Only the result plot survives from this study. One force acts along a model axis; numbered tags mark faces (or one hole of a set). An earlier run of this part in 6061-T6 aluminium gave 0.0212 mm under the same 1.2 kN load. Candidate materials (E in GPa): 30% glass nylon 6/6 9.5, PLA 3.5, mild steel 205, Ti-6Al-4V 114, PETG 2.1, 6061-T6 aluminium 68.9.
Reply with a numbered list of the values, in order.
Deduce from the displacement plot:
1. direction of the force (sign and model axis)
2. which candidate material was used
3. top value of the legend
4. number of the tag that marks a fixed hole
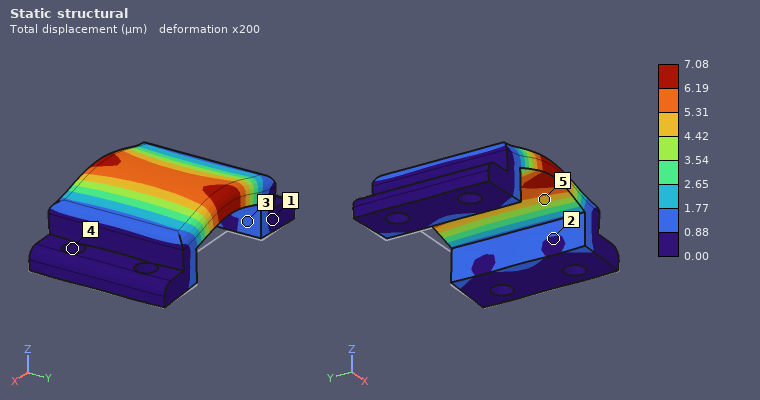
1. +Z
2. mild steel
3. 7.08 µm
4. 4
